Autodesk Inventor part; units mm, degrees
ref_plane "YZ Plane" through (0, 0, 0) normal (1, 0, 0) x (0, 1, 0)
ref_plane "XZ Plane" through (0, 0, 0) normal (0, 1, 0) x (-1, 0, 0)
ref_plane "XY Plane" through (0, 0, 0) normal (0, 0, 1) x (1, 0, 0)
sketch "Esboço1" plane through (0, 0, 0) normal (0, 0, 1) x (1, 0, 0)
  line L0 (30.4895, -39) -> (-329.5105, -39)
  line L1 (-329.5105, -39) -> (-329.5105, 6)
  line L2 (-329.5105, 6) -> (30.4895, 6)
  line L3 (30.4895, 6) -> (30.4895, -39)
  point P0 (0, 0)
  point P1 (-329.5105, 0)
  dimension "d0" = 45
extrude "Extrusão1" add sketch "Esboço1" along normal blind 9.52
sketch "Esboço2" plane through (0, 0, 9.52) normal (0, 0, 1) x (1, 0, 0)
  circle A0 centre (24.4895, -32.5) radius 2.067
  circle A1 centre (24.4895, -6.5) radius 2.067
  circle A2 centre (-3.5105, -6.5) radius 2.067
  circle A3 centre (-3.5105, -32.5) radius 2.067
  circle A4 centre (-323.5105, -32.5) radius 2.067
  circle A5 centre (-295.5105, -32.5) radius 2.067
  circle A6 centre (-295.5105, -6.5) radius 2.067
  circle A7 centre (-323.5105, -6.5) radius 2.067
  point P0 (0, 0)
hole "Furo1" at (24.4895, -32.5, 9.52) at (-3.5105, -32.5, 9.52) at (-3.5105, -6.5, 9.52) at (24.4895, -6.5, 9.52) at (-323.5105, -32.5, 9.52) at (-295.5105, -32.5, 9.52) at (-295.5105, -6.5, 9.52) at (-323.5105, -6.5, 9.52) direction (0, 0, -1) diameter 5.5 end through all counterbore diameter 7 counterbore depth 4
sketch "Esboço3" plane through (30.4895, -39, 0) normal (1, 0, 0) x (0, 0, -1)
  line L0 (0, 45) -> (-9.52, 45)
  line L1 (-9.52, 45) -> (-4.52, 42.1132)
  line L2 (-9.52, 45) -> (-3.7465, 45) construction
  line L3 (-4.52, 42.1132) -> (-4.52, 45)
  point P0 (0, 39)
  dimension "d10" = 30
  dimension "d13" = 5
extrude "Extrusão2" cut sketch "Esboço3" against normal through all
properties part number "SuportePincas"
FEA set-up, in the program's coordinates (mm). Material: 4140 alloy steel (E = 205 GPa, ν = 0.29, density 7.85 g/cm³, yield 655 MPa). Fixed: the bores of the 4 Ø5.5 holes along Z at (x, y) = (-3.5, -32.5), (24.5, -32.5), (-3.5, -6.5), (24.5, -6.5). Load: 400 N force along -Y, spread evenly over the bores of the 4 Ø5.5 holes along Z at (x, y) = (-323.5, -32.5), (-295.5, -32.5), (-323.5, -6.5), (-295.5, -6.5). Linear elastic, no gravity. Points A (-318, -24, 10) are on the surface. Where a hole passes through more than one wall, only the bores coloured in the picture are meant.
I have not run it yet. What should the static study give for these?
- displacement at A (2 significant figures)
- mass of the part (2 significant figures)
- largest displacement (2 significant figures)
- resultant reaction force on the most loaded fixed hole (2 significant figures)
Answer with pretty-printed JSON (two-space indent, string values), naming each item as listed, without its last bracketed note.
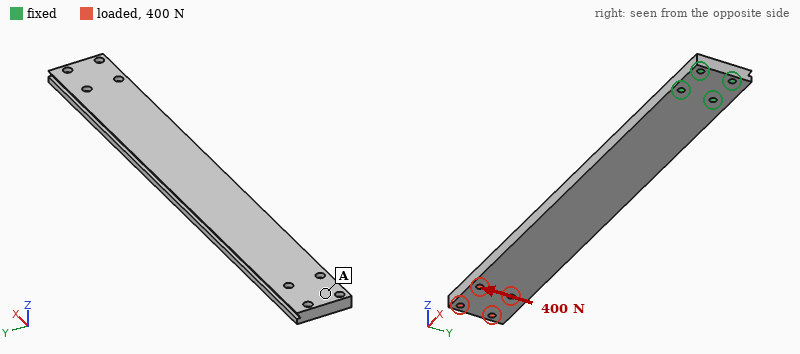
{
  "displacement at A": "0.30 mm",
  "mass of the part": "1.2 kg",
  "largest displacement": "0.32 mm",
  "resultant reaction force on the most loaded fixed hole": "3.5 kN"
}
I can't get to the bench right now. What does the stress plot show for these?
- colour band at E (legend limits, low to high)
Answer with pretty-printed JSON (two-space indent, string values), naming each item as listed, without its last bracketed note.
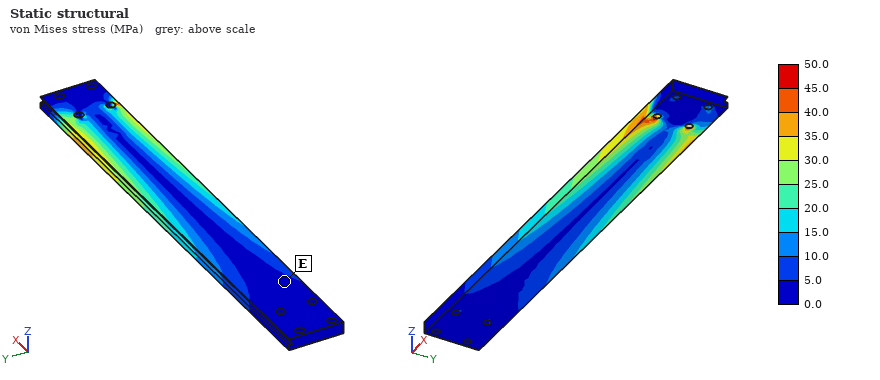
{
  "colour band at E": "0.0 to 5.0 MPa"
}
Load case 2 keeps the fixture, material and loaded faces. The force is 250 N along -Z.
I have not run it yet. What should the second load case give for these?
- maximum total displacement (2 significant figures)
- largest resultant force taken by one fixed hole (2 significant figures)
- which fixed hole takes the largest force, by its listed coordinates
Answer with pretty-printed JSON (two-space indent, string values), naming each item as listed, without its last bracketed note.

{
  "maximum total displacement": "4.1 mm",
  "largest resultant force taken by one fixed hole": "1.7 kN",
  "which fixed hole takes the largest force, by its listed coordinates": "(-3.5, -6.5)"
}
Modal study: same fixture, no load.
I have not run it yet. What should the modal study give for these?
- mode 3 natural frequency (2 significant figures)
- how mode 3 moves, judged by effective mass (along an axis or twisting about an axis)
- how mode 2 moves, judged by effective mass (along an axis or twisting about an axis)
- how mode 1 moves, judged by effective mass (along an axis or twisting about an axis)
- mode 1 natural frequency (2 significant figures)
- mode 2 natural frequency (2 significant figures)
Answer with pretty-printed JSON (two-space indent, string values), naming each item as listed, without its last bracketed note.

{
  "mode 3 natural frequency": "460 Hz",
  "how mode 3 moves, judged by effective mass": "along Z",
  "how mode 2 moves, judged by effective mass": "along Y",
  "how mode 1 moves, judged by effective mass": "along Z",
  "mode 1 natural frequency": "73 Hz",
  "mode 2 natural frequency": "330 Hz"
}
